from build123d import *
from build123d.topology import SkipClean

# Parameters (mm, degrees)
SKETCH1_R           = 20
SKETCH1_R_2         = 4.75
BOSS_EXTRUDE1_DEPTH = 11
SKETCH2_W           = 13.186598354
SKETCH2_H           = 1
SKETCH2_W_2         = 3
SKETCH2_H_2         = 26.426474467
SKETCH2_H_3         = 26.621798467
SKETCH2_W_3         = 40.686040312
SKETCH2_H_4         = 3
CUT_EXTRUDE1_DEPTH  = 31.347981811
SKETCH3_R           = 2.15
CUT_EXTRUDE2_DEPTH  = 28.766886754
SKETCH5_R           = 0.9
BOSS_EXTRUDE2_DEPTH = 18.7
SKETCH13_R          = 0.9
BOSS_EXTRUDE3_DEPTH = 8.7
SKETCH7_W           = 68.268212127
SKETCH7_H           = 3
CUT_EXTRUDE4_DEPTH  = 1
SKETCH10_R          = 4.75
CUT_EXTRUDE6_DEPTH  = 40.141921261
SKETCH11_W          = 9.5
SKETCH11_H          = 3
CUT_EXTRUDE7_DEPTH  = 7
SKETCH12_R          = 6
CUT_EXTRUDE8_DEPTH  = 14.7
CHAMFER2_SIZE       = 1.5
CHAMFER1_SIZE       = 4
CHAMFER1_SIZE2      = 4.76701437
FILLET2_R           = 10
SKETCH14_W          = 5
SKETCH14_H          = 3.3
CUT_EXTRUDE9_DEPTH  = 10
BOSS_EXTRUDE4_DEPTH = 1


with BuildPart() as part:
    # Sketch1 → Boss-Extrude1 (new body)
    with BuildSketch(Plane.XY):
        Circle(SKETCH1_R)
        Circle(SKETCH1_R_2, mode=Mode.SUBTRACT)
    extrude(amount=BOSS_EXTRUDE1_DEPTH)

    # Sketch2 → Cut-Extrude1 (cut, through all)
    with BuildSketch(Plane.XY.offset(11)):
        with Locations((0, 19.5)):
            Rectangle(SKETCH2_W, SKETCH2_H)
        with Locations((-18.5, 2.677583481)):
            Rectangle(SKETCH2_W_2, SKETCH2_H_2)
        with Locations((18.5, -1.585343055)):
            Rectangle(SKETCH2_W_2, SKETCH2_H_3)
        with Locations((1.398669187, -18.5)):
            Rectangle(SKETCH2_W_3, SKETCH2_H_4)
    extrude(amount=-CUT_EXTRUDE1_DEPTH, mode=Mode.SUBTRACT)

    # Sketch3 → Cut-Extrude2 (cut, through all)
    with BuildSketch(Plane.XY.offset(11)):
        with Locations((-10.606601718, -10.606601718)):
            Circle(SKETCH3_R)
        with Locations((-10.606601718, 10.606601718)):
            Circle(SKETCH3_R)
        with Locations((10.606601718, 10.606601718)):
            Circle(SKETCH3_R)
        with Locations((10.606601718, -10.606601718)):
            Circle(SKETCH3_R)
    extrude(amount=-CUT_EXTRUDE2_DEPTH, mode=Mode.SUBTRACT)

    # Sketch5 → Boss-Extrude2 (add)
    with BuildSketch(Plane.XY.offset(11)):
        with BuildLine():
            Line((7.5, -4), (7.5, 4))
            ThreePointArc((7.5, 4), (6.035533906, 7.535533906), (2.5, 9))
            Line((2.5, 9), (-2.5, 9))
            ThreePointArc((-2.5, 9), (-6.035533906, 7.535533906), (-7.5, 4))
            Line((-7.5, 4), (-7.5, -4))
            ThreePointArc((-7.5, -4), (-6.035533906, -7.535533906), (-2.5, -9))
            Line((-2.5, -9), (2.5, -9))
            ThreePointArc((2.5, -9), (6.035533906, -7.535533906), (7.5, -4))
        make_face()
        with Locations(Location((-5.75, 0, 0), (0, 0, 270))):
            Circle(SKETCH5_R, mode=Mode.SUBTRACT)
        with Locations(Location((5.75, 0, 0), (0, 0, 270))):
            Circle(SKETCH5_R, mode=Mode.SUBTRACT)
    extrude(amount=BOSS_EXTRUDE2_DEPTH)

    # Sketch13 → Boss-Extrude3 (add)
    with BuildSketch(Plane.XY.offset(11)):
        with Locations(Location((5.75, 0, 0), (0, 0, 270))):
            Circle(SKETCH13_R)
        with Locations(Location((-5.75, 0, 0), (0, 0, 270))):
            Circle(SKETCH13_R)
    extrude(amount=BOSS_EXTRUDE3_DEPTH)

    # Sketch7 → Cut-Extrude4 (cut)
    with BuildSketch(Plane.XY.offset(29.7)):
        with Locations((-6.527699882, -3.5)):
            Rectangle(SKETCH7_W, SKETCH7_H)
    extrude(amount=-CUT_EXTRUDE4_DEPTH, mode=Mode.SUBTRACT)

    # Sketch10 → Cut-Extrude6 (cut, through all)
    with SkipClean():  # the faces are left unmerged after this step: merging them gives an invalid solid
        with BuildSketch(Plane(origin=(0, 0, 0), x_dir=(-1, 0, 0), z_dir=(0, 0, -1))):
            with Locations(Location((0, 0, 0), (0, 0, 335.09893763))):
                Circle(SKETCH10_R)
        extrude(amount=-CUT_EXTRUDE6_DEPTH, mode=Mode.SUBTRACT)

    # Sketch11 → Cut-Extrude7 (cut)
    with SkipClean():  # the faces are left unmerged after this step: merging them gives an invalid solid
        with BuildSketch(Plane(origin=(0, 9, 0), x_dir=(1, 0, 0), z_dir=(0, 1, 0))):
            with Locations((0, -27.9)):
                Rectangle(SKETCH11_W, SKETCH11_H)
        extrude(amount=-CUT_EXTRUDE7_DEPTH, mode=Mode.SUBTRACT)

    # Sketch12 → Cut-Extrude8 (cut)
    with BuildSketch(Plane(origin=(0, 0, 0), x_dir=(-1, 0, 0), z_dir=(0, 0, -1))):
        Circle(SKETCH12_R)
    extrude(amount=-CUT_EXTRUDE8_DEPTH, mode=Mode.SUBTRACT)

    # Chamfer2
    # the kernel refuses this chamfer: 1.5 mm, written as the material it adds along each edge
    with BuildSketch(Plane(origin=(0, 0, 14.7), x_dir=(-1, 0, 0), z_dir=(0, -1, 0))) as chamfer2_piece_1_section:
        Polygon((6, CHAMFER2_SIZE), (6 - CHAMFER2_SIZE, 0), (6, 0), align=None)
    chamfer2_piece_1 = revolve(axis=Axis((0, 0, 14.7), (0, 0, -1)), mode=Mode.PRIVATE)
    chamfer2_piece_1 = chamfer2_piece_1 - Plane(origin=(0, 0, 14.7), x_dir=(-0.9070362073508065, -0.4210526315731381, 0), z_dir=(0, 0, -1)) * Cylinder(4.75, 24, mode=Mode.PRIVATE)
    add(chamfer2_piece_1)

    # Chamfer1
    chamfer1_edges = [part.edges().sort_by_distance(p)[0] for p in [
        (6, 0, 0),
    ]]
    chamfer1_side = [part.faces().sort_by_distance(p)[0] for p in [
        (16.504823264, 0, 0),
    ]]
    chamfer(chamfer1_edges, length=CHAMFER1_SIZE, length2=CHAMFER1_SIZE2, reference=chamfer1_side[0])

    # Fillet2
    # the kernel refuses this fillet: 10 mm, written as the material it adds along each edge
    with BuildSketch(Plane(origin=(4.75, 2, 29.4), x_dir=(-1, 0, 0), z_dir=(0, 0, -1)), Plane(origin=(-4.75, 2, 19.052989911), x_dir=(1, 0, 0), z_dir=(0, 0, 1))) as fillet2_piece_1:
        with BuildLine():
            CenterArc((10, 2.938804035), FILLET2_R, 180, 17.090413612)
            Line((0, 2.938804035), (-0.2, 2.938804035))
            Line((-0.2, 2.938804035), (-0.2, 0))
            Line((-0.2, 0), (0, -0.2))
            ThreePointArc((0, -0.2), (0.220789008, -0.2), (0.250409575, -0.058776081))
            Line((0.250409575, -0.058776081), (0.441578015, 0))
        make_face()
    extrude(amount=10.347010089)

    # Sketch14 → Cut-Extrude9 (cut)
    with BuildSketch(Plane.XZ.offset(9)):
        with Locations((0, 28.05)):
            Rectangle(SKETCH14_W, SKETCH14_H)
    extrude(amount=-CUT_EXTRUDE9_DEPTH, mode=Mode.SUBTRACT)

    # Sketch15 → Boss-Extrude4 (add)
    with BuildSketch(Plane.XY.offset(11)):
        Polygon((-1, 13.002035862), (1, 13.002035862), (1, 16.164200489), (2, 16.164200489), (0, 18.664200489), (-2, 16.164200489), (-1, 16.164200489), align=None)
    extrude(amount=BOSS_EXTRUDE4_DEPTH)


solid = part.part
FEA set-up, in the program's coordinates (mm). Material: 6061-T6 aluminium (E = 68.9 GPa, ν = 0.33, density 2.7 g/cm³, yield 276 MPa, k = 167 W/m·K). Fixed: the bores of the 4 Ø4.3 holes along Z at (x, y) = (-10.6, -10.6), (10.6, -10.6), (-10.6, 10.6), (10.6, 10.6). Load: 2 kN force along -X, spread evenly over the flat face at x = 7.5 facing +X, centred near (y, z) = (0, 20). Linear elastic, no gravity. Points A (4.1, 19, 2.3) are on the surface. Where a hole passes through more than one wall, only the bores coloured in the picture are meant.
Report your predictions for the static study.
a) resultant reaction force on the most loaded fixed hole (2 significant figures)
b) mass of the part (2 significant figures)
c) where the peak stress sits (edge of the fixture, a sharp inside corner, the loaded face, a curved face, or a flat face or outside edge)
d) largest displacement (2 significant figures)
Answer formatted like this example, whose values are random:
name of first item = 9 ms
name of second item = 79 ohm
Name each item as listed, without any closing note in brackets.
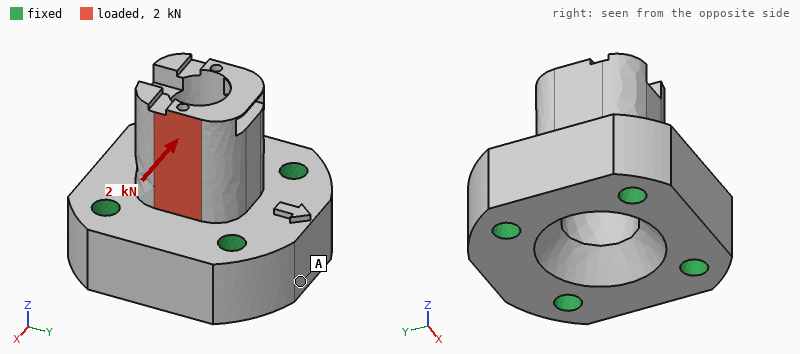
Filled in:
resultant reaction force on the most loaded fixed hole = 910 N
mass of the part = 35 g
where the peak stress sits = a curved face
largest displacement = 38 µm
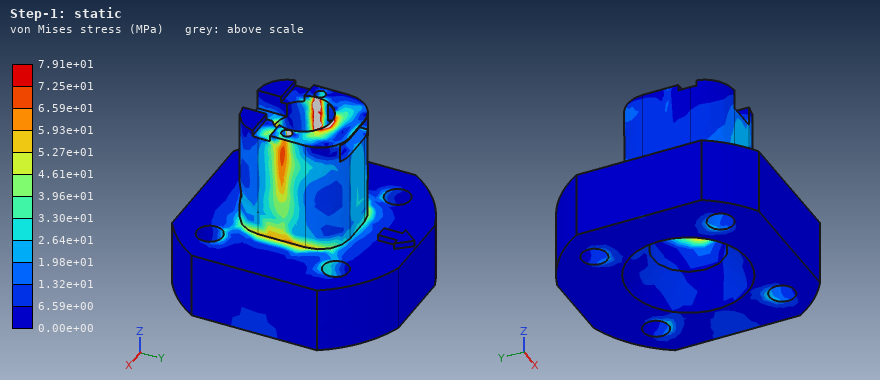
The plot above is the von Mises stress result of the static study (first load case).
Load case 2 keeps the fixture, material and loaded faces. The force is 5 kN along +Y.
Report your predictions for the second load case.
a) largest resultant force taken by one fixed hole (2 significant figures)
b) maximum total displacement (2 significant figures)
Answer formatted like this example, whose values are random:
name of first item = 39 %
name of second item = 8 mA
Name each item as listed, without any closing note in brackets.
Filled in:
largest resultant force taken by one fixed hole = 2.5 kN
maximum total displacement = 69 µm
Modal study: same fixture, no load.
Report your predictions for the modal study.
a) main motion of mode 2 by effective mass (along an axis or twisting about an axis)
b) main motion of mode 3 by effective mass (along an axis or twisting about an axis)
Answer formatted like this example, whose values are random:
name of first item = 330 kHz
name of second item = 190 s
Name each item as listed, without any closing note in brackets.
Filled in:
main motion of mode 2 by effective mass = along X
main motion of mode 3 by effective mass = along Y
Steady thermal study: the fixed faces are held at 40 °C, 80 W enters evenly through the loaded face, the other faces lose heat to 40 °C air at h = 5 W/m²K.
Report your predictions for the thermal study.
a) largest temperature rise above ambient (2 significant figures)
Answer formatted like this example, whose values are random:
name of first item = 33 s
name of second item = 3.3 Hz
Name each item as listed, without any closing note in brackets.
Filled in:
largest temperature rise above ambient = 66 K
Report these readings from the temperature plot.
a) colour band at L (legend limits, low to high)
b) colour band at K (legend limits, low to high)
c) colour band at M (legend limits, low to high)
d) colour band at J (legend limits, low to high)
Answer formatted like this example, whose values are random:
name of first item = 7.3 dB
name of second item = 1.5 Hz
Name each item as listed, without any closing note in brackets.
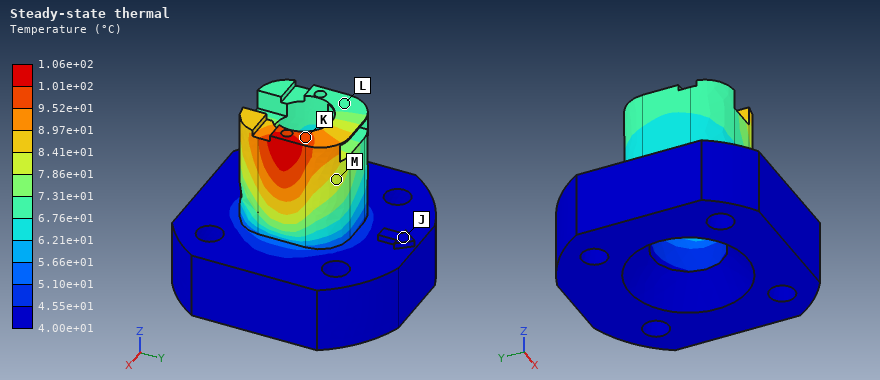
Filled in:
colour band at L = 6.76e+01 to 7.31e+01 °C
colour band at K = 9.52e+01 to 1.01e+02 °C
colour band at M = 7.86e+01 to 8.41e+01 °C
colour band at J = 4.00e+01 to 4.55e+01 °C
